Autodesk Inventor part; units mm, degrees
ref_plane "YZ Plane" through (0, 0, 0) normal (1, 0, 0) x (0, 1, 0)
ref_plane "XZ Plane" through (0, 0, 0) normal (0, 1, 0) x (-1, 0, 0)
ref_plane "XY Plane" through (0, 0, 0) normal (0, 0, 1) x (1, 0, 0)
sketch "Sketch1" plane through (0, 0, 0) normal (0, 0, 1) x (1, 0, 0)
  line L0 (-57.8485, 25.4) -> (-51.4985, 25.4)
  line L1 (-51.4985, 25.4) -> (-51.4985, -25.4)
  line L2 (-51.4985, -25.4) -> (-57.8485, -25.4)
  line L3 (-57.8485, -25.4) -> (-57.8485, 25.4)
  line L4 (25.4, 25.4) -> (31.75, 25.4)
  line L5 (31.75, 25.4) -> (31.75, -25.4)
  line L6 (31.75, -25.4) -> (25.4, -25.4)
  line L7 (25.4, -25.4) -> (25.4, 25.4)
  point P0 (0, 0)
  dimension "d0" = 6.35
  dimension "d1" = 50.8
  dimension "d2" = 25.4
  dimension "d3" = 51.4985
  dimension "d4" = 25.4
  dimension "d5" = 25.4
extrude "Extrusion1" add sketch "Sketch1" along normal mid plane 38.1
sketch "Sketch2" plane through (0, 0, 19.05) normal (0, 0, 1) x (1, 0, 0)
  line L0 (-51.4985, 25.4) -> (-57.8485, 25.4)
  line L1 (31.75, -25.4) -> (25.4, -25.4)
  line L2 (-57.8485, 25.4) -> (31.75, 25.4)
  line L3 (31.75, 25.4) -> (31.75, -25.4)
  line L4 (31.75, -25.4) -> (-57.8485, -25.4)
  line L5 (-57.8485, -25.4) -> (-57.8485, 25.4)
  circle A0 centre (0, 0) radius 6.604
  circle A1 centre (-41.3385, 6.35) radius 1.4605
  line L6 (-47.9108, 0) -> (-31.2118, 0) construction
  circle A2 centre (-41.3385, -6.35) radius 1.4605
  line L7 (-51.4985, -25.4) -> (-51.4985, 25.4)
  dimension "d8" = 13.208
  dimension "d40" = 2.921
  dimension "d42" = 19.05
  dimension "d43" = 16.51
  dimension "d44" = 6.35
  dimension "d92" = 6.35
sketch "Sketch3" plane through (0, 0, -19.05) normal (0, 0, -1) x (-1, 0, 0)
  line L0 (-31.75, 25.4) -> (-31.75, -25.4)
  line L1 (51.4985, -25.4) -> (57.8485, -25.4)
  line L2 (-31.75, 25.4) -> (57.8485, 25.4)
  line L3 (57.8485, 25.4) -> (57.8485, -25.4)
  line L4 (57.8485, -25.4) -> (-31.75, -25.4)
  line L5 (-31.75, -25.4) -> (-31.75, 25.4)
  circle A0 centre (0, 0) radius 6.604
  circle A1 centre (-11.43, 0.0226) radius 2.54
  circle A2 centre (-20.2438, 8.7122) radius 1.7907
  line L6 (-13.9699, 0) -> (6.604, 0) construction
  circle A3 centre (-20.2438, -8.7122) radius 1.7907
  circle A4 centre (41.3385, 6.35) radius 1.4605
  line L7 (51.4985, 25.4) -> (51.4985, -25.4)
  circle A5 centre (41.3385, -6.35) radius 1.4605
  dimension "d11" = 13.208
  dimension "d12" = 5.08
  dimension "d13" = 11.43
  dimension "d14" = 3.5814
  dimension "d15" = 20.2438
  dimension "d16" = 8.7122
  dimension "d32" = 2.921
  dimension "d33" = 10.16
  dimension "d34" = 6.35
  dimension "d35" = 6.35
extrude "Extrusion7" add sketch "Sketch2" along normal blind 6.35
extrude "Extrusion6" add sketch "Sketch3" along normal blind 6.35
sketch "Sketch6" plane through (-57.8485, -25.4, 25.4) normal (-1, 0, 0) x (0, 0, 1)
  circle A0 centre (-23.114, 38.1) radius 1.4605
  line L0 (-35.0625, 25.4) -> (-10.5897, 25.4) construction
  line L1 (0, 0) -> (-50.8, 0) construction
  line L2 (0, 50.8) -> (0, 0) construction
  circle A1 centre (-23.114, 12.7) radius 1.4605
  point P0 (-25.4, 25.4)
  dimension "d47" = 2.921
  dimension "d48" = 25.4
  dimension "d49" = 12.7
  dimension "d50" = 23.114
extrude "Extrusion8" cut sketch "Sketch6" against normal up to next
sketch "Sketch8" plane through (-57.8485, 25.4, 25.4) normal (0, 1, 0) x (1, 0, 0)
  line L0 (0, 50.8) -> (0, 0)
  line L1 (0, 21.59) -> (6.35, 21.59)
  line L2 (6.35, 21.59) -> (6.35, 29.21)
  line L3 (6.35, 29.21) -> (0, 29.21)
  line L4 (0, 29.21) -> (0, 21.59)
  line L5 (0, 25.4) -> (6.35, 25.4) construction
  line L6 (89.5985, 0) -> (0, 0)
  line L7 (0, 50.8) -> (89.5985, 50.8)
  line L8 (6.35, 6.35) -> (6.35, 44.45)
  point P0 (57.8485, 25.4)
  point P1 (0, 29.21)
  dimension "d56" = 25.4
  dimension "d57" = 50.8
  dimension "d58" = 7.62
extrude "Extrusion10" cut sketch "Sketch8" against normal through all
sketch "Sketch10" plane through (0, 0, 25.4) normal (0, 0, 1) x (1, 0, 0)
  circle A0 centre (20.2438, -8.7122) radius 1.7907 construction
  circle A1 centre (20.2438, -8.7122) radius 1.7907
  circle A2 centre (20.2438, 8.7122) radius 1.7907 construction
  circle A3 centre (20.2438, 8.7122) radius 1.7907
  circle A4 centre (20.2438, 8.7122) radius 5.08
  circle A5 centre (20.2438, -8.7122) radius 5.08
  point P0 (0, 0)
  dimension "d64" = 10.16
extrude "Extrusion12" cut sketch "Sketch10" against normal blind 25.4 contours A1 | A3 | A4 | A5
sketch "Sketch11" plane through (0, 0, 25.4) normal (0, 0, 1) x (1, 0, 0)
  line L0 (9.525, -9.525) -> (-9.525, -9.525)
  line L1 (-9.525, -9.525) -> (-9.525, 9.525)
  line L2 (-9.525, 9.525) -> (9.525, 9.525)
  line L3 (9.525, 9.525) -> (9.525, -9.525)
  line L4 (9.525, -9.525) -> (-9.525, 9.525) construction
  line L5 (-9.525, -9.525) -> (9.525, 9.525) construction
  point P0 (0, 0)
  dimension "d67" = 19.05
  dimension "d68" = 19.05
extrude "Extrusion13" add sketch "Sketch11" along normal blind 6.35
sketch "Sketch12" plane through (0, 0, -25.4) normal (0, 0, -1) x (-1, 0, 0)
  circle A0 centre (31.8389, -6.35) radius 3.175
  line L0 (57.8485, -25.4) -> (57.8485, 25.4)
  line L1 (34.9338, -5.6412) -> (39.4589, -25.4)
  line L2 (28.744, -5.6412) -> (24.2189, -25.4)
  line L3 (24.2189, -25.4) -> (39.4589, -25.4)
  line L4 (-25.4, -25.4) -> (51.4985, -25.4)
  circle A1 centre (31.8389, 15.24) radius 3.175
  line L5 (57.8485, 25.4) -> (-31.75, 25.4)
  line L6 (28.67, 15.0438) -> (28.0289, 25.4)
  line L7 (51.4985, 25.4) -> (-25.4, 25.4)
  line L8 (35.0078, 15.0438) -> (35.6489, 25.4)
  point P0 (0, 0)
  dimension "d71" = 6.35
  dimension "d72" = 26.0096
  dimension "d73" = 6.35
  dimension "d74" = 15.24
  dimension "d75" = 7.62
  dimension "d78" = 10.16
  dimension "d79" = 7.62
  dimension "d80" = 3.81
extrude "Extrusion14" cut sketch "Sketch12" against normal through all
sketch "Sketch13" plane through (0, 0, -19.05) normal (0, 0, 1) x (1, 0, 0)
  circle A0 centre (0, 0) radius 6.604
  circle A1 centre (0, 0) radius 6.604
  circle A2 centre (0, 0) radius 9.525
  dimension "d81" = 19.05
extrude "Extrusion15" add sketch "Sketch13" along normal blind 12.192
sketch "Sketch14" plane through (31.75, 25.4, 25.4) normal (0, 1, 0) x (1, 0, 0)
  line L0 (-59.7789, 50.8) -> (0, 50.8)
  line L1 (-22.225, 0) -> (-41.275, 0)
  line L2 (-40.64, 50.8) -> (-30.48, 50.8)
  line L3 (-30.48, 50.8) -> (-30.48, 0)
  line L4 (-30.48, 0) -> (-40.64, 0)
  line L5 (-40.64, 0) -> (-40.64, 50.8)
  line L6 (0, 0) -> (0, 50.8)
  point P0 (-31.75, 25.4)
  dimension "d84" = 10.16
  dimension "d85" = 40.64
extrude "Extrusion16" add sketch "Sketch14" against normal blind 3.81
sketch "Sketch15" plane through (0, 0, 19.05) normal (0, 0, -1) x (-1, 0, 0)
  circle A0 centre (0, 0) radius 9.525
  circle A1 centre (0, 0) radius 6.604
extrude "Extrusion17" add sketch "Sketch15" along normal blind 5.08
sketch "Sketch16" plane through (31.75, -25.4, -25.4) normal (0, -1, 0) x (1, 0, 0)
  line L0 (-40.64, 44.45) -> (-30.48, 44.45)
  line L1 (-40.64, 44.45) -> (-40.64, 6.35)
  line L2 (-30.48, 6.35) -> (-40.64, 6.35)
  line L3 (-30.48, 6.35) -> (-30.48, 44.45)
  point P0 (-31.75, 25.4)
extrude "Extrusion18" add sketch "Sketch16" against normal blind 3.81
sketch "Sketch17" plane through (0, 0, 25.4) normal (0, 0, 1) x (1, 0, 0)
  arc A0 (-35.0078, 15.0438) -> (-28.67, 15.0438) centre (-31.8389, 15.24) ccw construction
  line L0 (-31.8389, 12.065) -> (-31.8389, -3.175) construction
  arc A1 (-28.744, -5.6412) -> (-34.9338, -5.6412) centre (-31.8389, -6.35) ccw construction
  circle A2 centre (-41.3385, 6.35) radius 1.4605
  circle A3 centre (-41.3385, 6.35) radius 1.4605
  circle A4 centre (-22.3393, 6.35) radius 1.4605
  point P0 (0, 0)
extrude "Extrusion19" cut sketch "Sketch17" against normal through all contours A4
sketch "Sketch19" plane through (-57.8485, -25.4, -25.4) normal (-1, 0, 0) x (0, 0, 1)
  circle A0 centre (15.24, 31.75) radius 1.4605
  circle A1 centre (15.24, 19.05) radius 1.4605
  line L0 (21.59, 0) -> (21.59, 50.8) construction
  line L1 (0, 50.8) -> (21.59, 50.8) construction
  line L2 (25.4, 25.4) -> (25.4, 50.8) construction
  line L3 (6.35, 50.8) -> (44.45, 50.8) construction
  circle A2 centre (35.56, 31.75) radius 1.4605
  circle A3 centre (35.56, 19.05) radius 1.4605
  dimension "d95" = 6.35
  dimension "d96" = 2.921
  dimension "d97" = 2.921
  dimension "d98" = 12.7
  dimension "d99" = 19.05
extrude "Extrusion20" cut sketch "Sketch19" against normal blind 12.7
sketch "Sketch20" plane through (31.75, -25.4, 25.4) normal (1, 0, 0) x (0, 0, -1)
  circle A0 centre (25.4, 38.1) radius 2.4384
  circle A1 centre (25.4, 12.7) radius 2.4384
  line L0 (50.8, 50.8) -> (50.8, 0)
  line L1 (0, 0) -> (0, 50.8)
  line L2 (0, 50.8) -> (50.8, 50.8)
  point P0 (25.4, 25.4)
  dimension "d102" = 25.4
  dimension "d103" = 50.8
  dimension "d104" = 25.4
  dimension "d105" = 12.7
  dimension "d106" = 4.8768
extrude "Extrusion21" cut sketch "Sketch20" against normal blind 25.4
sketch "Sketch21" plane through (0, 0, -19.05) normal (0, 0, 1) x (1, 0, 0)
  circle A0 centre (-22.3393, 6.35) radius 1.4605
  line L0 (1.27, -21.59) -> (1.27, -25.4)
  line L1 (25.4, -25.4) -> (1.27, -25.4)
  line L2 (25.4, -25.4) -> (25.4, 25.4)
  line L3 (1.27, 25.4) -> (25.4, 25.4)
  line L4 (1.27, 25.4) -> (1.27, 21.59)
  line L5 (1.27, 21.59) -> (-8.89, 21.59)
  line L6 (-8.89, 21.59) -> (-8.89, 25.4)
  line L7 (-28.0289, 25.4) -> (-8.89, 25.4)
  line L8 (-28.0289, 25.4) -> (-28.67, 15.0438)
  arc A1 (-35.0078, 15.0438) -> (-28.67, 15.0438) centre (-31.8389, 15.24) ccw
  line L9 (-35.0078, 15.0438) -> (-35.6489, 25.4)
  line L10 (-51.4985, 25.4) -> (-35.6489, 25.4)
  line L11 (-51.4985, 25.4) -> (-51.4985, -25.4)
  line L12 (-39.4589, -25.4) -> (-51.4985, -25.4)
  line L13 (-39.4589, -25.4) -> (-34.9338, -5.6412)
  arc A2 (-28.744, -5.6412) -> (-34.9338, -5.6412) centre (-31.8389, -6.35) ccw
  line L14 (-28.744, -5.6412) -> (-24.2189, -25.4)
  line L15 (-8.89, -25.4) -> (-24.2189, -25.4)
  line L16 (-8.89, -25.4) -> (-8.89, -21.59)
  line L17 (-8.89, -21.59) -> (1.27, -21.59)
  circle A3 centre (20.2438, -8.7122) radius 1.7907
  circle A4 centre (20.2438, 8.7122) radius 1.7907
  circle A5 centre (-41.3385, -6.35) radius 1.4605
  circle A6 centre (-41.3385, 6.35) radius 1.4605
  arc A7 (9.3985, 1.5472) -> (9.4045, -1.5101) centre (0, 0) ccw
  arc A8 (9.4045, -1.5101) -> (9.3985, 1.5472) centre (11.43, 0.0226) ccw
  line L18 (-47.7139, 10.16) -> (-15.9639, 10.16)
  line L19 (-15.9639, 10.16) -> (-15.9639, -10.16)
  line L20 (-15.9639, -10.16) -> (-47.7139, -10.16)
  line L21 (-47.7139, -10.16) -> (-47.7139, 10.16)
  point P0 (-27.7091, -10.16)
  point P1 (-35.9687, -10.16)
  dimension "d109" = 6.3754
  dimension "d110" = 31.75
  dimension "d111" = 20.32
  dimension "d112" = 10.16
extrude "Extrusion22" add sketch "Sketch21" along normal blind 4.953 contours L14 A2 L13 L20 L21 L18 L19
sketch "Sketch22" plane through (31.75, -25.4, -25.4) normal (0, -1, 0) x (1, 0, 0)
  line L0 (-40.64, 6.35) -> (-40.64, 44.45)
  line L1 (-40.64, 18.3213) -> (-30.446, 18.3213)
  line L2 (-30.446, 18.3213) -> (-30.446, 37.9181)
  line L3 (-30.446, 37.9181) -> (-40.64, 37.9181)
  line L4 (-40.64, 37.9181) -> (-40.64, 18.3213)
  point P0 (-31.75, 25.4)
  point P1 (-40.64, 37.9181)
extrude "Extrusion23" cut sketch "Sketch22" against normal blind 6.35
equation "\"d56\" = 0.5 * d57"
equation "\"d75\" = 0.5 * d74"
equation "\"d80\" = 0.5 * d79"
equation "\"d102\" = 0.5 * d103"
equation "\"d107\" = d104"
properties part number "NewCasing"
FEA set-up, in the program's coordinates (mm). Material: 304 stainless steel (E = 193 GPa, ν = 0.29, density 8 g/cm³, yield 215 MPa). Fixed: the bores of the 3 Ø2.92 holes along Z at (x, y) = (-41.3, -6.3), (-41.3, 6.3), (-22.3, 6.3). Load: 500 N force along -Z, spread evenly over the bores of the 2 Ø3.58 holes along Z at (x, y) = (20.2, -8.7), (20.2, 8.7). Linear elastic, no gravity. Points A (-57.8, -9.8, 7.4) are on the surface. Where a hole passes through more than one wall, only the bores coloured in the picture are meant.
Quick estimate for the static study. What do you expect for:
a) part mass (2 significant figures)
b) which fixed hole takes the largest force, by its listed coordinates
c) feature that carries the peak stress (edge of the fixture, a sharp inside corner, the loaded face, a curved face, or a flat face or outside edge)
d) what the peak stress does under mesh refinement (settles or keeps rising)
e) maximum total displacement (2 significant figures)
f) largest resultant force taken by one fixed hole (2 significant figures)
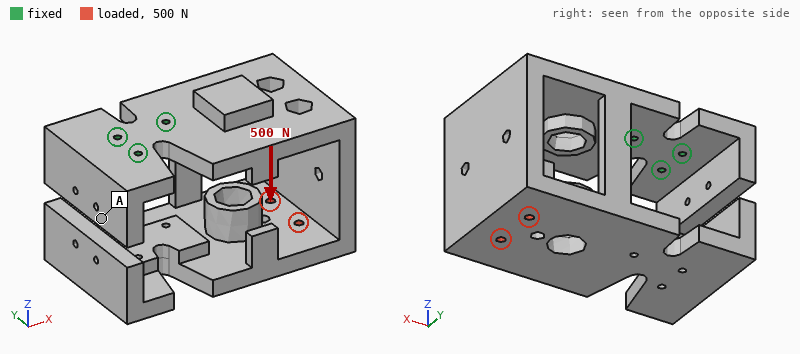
660 g
(-22.3, 6.3)
edge of the fixture
keeps rising
0.18 mm
1.1 kN
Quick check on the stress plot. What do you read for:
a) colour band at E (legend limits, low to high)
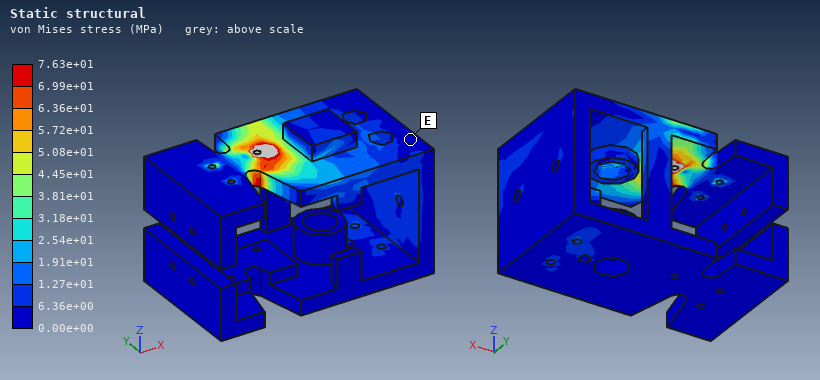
0.00e+00 to 6.36e+00 MPa
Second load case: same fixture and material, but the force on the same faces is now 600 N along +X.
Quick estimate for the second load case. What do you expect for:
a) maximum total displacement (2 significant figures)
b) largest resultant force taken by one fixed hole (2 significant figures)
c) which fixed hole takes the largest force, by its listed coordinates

0.39 mm
840 N
(-22.3, 6.3)
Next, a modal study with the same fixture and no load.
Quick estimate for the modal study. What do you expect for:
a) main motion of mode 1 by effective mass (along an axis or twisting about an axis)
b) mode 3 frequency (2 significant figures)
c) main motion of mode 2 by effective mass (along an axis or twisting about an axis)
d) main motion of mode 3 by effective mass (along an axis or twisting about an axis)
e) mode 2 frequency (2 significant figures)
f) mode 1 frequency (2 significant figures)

along X
680 Hz
along Y
along Z
380 Hz
350 Hz
